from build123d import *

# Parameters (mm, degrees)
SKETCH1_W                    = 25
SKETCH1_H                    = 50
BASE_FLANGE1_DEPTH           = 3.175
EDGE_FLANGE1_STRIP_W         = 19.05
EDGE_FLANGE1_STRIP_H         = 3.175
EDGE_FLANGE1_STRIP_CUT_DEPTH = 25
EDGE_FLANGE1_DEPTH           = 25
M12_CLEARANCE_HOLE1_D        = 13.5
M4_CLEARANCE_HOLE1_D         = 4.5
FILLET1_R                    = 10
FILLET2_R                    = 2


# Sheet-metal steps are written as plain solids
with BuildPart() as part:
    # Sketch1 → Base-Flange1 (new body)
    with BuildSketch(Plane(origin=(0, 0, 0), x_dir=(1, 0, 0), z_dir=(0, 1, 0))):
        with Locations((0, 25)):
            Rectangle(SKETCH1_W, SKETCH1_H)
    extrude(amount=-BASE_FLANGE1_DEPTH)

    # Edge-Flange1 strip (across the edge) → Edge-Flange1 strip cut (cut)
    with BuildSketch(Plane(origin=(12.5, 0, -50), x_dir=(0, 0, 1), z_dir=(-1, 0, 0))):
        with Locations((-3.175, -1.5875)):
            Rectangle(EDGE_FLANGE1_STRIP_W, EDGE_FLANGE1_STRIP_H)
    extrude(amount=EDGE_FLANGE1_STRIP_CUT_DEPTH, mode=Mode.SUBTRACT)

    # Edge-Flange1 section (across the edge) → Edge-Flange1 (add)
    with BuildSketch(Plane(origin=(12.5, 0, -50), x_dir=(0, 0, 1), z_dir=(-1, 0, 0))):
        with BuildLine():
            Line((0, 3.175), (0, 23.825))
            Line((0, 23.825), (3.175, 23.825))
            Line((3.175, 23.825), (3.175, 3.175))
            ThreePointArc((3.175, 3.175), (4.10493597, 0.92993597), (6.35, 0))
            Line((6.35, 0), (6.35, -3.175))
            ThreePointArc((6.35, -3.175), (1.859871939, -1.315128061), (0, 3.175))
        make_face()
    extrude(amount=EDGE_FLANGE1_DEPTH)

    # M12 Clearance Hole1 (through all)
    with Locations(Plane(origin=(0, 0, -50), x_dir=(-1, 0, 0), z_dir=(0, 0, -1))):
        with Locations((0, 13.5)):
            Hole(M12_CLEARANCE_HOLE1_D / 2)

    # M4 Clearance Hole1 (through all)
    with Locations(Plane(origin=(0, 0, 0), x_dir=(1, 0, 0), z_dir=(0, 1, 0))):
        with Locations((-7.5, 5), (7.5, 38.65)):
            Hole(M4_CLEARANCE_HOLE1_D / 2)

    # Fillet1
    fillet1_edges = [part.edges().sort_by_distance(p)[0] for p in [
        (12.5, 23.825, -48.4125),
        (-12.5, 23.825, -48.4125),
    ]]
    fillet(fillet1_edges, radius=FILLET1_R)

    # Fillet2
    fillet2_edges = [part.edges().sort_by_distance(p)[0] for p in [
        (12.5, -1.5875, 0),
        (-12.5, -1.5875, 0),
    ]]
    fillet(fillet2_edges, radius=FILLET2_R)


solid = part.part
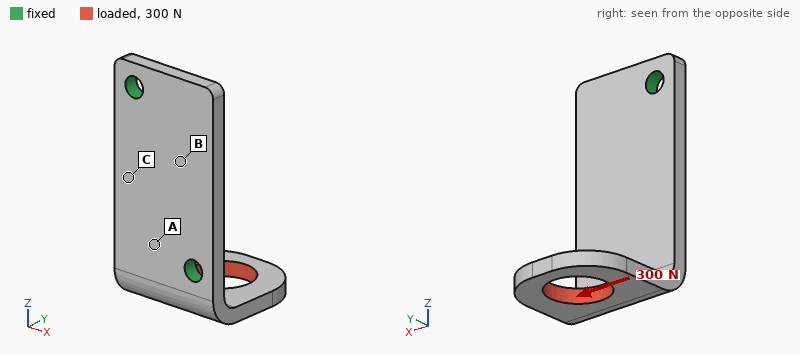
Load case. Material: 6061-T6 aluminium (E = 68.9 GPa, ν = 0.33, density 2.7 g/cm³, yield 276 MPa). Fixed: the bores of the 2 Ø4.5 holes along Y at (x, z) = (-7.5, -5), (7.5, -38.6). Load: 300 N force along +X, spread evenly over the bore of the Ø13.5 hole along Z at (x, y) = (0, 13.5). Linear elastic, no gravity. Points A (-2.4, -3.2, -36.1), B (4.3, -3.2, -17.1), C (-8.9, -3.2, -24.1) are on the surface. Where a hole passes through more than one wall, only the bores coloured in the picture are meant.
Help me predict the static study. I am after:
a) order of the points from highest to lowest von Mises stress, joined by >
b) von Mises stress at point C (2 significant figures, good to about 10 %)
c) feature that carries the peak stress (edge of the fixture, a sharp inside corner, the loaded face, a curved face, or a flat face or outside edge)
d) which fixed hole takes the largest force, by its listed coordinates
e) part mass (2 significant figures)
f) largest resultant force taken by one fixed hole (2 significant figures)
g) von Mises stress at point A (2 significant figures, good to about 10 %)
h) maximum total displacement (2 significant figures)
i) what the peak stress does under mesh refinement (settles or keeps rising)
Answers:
A > C > B
24 MPa
edge of the fixture
(7.5, -38.6)
14 g
330 N
39 MPa
0.18 mm
keeps rising
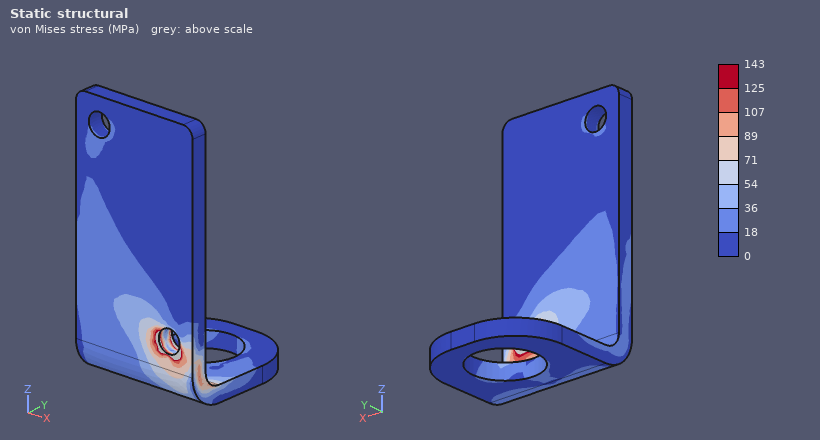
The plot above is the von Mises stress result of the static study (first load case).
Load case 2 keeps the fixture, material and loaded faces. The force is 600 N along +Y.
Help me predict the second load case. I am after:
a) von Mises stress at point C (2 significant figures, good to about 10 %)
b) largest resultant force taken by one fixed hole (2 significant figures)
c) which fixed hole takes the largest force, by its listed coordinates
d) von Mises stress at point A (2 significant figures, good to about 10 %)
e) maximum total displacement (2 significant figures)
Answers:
24 MPa
640 N
(7.5, -38.6)
62 MPa
0.27 mm
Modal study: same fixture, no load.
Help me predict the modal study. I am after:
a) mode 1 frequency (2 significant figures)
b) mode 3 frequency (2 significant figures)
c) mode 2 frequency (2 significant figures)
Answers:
3100 Hz
8000 Hz
4100 Hz
